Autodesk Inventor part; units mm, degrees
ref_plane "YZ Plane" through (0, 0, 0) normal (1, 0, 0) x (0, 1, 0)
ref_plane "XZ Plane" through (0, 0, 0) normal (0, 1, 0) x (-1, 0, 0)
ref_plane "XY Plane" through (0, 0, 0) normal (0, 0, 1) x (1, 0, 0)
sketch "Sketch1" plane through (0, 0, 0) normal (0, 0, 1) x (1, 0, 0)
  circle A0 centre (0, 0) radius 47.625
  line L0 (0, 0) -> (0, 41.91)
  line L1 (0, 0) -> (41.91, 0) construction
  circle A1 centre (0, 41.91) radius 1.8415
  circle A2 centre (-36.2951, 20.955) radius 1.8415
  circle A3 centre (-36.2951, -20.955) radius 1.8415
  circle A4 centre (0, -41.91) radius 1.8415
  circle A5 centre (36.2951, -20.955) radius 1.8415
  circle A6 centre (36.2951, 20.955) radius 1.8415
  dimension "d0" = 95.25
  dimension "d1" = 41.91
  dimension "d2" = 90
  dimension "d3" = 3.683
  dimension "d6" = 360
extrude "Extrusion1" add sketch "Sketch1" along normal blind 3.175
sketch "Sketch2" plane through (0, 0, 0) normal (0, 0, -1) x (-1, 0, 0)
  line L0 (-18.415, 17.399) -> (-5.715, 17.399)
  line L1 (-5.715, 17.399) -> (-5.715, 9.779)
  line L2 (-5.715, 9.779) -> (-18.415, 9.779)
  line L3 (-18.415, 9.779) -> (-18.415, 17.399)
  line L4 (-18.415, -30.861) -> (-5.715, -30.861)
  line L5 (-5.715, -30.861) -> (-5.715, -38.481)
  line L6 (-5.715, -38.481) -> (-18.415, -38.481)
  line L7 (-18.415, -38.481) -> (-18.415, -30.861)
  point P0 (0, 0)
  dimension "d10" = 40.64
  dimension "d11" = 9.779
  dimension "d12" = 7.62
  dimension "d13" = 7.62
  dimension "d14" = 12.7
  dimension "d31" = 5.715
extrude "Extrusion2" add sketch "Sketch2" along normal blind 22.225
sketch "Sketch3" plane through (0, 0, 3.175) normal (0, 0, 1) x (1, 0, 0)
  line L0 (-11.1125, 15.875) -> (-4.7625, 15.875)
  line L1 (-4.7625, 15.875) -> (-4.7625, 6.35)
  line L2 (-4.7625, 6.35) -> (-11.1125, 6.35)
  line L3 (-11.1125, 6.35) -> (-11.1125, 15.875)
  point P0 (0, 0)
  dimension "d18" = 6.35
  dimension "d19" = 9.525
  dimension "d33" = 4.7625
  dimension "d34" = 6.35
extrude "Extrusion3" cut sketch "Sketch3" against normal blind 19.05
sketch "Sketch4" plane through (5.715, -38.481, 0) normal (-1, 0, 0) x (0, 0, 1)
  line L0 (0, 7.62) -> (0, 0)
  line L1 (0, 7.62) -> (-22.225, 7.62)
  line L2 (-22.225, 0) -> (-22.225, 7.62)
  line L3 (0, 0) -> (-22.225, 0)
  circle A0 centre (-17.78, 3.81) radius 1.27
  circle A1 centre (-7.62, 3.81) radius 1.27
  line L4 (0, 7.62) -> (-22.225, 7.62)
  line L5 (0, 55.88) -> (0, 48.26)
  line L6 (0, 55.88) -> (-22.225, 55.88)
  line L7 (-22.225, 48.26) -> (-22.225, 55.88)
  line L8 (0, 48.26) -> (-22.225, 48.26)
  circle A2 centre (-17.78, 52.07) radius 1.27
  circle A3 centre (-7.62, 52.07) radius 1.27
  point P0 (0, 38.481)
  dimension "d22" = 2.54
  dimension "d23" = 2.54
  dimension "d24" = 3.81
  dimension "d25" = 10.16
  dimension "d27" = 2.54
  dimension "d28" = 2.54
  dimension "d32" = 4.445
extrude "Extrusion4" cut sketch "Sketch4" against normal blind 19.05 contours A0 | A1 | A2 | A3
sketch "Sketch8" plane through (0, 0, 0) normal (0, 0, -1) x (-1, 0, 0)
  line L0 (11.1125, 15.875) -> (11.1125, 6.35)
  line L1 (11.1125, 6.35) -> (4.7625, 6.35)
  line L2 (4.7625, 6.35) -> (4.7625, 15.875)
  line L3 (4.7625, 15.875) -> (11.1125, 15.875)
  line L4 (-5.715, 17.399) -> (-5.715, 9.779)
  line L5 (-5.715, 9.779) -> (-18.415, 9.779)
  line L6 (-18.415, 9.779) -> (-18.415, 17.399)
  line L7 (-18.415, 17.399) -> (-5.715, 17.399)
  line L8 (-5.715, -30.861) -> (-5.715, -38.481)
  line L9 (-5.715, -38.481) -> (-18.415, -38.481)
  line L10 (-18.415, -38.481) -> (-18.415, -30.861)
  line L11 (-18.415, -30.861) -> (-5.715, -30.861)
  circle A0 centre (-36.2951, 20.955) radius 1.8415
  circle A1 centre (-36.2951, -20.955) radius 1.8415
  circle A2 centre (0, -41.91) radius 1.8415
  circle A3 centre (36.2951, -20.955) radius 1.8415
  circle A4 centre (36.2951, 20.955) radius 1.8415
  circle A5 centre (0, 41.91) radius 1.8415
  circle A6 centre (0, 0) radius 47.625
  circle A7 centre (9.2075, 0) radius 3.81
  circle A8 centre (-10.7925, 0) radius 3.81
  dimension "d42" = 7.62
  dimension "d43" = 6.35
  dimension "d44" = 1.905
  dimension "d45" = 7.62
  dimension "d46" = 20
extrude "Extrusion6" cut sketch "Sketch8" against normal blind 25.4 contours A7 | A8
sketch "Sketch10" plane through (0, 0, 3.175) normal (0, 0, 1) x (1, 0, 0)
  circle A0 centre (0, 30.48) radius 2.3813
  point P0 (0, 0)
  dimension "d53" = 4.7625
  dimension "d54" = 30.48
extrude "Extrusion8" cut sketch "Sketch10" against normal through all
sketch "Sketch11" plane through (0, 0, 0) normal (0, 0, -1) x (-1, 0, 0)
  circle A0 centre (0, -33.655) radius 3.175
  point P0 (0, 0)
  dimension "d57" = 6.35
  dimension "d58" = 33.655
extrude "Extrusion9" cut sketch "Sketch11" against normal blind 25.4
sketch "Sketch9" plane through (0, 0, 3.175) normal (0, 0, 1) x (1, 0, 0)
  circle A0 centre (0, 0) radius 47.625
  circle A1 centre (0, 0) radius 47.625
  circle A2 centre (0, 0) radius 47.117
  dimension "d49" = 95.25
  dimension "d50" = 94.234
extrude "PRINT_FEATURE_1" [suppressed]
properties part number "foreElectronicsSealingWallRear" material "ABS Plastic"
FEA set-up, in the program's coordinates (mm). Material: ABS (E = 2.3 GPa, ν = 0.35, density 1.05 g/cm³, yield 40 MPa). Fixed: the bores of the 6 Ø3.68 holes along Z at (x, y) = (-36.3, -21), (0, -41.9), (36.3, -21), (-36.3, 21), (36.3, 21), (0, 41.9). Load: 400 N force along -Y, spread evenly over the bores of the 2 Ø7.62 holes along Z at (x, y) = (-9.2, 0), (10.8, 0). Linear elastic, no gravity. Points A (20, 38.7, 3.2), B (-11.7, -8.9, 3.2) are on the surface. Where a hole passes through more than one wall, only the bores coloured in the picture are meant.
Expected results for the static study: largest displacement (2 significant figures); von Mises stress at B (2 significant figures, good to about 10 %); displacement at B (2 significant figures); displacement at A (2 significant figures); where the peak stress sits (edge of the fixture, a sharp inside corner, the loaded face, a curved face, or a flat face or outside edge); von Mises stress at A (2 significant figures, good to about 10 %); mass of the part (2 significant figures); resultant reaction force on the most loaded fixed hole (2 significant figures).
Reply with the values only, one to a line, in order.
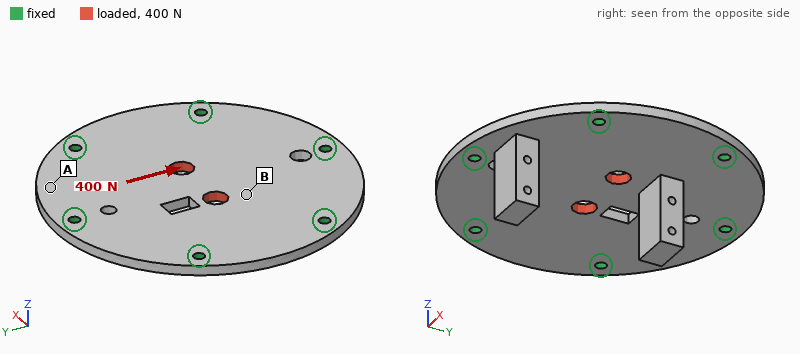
41 µm
1.9 MPa
24 µm
14 µm
a flat face or outside edge
0.66 MPa
27 g
86 N
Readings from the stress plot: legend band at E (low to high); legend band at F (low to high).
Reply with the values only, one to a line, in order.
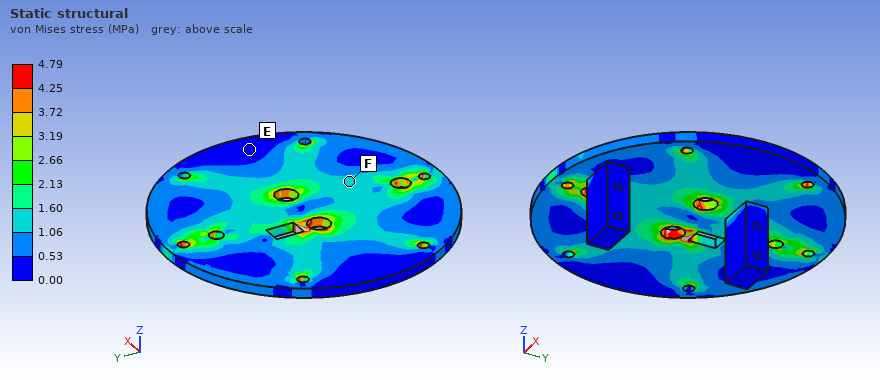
0.00 to 0.53 MPa
1.06 to 1.60 MPa
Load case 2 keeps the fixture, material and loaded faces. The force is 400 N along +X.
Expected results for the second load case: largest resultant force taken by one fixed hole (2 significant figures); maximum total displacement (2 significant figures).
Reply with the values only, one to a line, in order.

95 N
41 µm
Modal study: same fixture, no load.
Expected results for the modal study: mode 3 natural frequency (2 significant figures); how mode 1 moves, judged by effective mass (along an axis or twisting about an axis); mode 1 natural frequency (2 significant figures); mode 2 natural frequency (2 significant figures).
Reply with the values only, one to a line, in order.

1500 Hz
along Z
890 Hz
1400 Hz
